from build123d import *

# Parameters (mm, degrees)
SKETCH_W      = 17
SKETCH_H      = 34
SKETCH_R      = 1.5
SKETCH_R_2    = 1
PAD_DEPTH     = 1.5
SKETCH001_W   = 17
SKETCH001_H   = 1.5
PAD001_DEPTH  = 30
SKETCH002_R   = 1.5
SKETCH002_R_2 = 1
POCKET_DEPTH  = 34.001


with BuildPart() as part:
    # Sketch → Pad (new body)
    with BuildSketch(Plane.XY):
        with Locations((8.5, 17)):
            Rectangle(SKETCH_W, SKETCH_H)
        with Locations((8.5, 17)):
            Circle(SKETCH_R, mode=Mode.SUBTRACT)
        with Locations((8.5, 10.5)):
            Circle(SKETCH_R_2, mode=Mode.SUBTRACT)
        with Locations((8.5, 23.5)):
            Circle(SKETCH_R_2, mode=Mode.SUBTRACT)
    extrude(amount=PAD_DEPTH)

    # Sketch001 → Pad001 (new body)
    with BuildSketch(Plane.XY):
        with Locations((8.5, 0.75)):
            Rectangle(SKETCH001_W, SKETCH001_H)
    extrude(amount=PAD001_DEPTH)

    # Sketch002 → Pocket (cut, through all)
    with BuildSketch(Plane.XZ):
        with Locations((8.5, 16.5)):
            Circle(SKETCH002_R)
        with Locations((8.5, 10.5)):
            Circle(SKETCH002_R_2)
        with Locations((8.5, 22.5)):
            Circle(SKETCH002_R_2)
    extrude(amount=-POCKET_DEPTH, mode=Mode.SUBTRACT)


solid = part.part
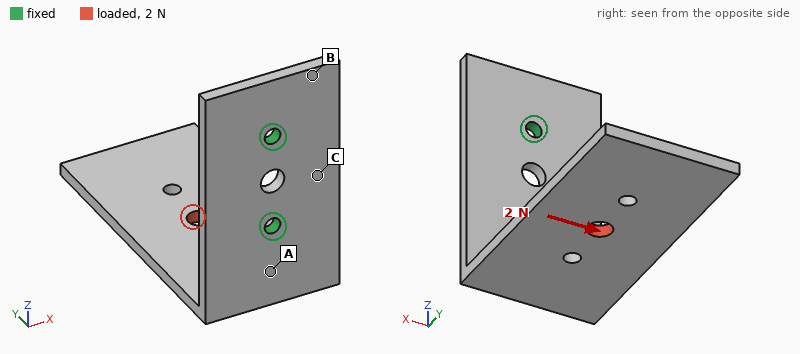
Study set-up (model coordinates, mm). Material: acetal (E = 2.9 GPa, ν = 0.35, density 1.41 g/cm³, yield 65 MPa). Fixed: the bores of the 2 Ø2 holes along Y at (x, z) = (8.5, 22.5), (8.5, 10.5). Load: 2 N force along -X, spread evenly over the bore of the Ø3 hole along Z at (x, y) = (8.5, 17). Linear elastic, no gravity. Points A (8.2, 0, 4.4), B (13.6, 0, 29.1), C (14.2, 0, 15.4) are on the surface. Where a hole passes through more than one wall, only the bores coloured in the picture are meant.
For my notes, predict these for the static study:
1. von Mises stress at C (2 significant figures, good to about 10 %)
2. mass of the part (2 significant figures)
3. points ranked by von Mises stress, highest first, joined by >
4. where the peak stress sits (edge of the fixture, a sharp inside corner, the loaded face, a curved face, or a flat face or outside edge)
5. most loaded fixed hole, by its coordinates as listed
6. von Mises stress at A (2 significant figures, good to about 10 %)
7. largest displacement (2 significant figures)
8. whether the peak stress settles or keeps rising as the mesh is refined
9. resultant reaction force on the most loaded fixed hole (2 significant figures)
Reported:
1.6 MPa
2.2 g
A > C > B
edge of the fixture
(8.5, 10.5)
3.4 MPa
0.47 mm
keeps rising
3.3 N
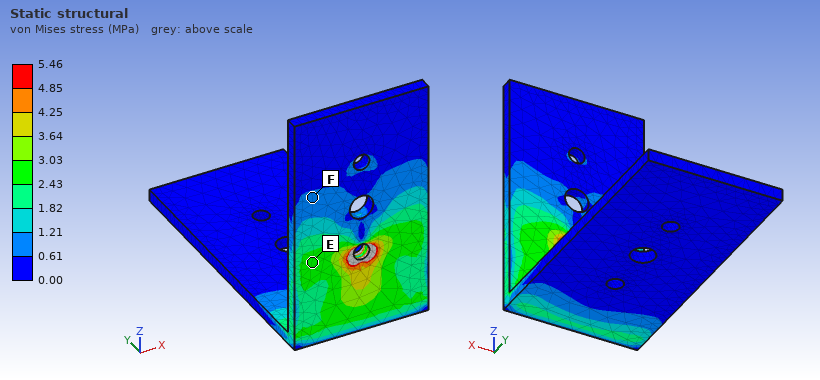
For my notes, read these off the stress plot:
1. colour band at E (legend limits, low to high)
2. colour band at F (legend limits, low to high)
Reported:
2.43 to 3.03 MPa
0.61 to 1.21 MPa
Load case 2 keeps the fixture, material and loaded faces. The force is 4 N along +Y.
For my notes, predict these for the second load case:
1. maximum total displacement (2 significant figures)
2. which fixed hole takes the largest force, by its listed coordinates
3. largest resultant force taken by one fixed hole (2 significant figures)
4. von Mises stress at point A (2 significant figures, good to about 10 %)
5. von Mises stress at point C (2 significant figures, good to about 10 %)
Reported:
0.49 mm
(8.5, 10.5)
5.1 N
2.1 MPa
0.82 MPa
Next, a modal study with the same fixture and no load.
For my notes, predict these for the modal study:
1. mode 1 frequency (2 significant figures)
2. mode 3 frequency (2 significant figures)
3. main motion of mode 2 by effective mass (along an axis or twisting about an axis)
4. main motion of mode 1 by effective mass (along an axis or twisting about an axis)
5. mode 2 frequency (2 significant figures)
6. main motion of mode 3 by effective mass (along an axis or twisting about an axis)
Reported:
220 Hz
1100 Hz
along X
along Z
360 Hz
along Y
